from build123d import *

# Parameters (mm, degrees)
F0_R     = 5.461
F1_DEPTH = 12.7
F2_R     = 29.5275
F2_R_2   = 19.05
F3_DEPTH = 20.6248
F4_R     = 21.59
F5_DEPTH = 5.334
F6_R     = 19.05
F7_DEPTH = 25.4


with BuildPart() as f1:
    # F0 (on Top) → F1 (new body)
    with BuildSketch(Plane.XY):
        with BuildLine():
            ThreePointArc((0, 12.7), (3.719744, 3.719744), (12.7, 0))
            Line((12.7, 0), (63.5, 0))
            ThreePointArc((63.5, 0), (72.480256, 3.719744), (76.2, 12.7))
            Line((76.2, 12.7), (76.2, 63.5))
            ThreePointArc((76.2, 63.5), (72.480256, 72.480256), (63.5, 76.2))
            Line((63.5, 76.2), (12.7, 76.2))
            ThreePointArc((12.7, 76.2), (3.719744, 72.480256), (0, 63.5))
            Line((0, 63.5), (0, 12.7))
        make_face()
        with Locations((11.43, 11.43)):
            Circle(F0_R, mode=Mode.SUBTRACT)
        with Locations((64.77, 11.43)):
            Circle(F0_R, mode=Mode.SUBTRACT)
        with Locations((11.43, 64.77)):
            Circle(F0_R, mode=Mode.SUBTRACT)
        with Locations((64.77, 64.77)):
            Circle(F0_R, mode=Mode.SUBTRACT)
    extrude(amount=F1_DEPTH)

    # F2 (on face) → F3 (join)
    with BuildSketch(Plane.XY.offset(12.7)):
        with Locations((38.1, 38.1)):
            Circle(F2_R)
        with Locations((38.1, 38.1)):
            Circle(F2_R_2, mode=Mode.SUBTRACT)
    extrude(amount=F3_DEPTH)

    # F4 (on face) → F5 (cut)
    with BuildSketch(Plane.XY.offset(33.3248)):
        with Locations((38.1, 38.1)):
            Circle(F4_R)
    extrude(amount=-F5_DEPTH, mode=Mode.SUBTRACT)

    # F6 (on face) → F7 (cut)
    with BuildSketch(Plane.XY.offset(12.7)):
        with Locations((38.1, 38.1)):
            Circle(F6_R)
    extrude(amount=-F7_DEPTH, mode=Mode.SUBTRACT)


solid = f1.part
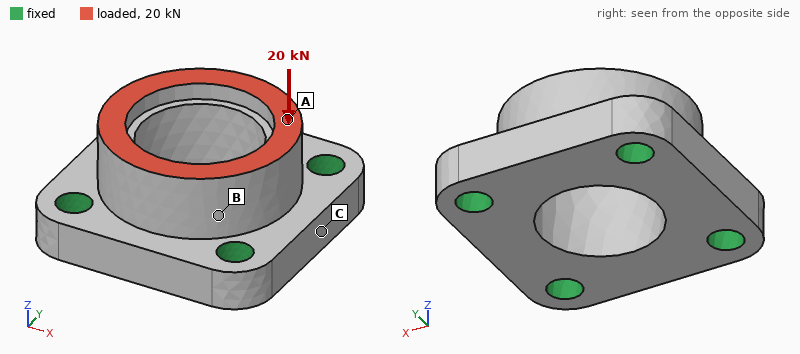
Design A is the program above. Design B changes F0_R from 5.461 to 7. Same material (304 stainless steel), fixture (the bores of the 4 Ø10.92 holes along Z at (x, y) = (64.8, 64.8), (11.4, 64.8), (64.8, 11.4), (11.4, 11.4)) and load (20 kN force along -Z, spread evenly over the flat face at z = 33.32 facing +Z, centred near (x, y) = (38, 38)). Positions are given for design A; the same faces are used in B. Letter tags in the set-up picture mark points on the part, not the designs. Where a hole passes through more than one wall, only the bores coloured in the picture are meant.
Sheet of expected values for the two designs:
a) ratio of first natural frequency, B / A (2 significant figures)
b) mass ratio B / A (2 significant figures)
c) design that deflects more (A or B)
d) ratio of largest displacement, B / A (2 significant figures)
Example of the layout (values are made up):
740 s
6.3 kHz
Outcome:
1.1
0.96
A
0.85
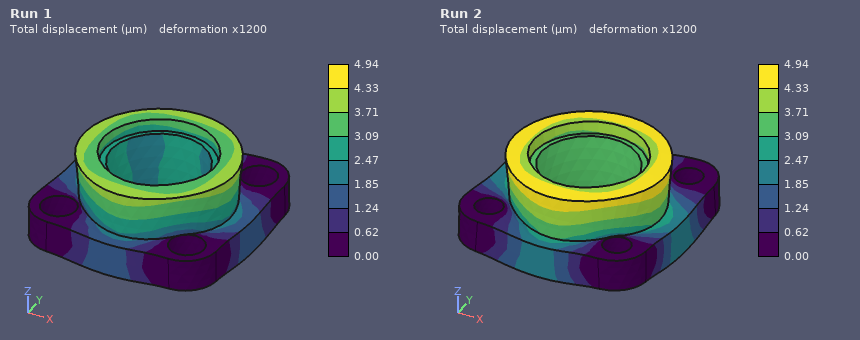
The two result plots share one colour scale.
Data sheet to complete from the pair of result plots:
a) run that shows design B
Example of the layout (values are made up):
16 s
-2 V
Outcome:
Run 1
